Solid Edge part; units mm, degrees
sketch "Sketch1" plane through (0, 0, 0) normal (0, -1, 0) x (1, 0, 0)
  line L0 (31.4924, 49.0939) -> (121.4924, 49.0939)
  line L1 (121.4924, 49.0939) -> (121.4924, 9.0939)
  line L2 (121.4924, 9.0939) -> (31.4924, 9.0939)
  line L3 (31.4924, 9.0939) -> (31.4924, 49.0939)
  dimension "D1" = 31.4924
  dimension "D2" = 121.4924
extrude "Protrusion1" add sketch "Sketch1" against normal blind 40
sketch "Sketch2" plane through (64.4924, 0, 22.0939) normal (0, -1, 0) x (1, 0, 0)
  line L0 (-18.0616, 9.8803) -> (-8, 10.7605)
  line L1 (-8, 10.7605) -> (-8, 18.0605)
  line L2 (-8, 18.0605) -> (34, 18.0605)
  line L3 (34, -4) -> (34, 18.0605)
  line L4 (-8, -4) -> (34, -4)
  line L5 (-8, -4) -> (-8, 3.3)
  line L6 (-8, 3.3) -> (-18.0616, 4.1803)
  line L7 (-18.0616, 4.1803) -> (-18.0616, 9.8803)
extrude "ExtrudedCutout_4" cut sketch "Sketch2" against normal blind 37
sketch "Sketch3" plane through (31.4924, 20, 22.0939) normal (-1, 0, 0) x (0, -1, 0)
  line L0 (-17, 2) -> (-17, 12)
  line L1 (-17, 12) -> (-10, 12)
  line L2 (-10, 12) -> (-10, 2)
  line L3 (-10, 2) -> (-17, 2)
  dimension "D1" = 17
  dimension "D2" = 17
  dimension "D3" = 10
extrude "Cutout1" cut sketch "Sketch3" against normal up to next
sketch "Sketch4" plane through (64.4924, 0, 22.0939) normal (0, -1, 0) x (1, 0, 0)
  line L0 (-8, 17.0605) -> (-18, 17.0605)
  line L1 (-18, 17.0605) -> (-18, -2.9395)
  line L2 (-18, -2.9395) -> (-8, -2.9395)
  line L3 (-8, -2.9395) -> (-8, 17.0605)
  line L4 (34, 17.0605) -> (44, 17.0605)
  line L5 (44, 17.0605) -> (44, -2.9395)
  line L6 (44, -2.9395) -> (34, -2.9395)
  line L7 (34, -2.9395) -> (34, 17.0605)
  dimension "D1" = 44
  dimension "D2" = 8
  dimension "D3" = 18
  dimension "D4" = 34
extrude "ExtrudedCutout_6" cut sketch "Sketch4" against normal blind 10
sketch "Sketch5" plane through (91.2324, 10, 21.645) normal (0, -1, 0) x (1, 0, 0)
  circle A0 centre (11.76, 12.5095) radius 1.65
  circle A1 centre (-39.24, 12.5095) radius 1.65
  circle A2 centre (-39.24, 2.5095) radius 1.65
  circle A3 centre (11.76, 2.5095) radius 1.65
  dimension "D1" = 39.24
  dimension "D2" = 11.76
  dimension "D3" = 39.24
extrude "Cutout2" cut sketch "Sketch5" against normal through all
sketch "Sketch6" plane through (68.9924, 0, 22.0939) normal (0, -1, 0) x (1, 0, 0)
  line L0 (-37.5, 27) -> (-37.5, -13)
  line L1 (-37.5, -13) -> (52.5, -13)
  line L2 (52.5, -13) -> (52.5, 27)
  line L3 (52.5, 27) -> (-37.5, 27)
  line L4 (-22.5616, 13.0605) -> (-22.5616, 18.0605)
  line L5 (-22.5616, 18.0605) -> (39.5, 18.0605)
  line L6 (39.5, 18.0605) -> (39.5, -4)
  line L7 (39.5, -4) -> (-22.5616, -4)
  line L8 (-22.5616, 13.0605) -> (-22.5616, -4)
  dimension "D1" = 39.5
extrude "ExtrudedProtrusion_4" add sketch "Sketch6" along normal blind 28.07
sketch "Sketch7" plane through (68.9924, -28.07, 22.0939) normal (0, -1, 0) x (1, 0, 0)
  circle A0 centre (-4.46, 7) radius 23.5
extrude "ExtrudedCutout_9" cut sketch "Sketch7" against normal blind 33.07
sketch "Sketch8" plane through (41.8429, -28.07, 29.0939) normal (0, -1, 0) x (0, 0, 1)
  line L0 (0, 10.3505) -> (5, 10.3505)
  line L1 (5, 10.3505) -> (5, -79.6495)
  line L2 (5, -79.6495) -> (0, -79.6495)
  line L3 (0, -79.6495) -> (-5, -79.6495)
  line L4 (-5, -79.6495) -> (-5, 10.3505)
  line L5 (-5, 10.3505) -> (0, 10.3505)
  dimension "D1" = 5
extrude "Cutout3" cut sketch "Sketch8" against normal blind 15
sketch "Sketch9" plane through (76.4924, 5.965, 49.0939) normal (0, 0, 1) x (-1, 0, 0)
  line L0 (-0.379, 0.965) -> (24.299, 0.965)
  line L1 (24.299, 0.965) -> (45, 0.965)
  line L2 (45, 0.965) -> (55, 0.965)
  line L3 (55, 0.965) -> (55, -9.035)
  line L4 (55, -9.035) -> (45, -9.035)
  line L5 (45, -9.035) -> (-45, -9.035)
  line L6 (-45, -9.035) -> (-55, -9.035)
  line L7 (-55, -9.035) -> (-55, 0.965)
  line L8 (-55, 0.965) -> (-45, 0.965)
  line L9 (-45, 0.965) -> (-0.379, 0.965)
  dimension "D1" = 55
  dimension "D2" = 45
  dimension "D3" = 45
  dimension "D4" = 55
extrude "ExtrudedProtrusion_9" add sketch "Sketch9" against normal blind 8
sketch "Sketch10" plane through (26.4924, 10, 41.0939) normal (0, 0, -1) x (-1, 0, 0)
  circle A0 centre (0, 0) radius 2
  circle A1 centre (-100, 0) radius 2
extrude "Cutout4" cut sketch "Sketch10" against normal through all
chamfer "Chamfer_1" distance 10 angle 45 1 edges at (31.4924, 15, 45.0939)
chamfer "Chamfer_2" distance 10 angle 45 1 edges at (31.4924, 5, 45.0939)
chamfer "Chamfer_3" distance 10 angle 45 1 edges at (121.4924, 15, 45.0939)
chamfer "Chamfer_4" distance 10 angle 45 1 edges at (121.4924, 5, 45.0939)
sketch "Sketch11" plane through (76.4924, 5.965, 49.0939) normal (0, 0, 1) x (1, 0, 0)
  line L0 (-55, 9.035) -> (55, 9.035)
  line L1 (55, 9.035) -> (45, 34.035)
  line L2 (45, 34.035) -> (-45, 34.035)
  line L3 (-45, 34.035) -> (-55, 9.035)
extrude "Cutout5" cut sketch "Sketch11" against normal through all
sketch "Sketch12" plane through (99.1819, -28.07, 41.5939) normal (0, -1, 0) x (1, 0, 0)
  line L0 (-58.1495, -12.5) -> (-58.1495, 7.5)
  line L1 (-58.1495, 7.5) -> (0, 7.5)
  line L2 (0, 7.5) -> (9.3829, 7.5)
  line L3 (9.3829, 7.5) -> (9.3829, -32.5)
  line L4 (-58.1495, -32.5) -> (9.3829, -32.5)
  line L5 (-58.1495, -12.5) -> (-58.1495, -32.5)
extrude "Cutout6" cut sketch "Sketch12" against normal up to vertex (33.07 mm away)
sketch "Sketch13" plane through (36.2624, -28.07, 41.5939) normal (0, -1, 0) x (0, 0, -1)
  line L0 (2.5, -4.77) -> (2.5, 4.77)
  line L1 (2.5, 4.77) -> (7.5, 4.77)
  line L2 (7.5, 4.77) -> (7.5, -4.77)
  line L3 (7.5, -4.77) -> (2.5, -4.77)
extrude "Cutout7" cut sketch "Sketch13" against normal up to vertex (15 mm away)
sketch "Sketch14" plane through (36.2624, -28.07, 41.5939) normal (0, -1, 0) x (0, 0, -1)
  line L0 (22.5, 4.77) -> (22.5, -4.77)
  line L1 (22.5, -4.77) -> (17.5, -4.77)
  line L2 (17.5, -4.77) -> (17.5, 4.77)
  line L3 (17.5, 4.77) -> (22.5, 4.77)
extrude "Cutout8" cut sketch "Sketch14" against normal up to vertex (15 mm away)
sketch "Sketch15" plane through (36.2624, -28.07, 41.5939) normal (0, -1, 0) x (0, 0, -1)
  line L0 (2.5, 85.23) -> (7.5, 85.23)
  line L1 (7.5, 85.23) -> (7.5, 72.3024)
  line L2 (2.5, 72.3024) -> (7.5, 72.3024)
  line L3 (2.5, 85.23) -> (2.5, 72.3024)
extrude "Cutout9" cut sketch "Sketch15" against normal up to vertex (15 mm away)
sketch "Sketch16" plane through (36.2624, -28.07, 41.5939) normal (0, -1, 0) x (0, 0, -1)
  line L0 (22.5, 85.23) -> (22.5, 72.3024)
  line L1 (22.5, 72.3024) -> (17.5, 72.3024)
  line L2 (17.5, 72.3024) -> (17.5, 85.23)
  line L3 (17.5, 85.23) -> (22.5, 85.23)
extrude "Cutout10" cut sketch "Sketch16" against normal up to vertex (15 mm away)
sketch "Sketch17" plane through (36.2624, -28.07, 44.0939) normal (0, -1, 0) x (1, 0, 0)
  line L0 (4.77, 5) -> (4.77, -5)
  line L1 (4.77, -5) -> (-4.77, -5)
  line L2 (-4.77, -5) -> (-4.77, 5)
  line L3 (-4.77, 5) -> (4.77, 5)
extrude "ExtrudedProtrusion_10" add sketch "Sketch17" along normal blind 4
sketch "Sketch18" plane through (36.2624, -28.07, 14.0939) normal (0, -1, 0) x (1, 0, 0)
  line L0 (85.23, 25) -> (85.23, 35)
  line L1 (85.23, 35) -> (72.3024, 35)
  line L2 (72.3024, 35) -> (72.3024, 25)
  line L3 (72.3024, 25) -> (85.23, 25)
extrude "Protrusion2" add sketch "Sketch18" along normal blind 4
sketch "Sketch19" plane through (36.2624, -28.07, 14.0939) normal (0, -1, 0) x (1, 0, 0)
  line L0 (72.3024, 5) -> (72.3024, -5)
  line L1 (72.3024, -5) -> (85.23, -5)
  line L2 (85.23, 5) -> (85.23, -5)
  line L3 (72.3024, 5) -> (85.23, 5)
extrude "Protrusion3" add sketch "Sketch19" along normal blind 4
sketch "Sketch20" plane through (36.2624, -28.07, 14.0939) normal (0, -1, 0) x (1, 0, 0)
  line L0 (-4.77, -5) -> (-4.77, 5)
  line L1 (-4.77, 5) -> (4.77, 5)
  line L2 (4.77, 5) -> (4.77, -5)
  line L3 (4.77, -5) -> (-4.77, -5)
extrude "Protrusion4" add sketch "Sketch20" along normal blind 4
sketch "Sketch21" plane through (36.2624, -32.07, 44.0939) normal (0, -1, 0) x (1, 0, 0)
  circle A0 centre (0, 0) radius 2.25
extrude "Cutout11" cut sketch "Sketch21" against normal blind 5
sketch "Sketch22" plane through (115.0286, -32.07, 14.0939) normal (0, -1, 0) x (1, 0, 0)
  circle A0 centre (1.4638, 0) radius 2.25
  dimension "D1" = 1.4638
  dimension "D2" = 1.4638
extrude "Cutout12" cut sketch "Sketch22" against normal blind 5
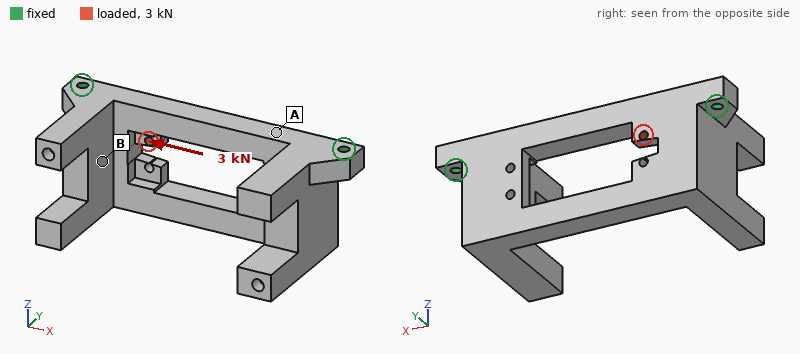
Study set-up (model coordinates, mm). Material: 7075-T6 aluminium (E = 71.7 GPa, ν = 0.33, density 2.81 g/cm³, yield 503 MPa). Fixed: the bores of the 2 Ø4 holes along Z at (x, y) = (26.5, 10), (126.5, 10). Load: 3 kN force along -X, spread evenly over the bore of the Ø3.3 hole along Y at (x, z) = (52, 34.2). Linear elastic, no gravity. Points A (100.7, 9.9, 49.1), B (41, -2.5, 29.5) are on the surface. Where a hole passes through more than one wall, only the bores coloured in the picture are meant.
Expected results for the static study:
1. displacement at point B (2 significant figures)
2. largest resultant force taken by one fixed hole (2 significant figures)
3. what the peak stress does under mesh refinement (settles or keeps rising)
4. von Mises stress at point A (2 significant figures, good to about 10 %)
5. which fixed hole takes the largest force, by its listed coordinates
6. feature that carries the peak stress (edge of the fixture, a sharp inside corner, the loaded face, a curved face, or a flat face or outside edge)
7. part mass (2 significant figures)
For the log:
9.9 µm
2.2 kN
keeps rising
26 MPa
(26.5, 10)
a sharp inside corner
140 g
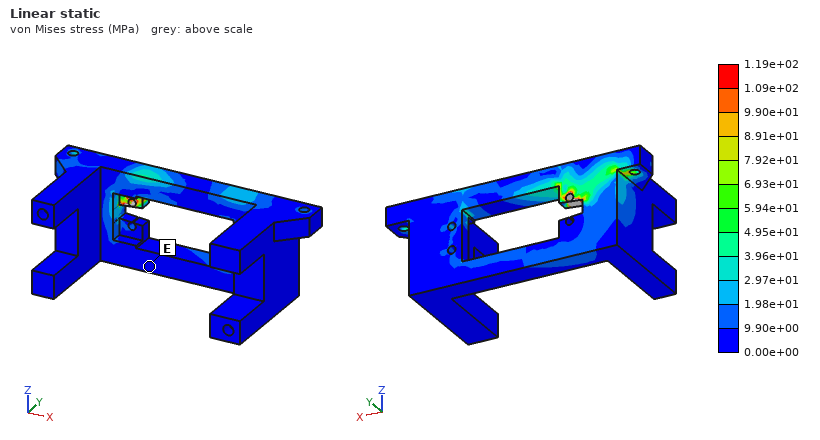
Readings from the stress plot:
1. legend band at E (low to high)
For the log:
0.00e+00 to 9.90e+00 MPa
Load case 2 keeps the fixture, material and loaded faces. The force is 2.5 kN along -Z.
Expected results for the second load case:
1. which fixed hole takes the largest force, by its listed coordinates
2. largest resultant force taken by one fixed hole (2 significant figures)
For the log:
(26.5, 10)
2.1 kN
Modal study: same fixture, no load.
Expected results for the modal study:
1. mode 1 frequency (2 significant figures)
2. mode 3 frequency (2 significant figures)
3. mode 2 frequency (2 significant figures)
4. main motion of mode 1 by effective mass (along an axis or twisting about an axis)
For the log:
1700 Hz
2800 Hz
2400 Hz
along Y
